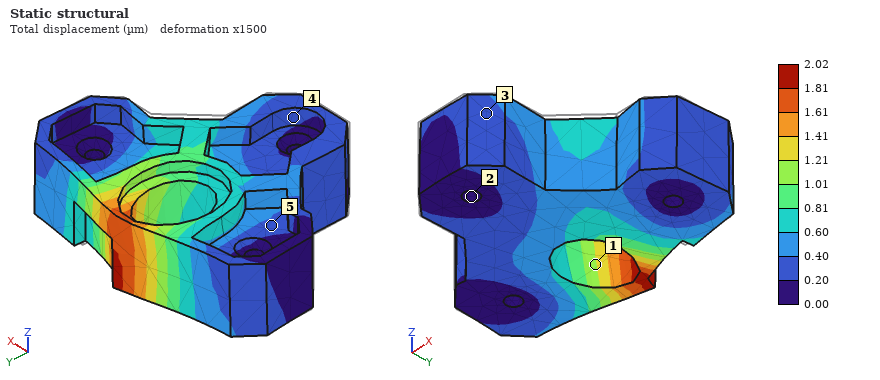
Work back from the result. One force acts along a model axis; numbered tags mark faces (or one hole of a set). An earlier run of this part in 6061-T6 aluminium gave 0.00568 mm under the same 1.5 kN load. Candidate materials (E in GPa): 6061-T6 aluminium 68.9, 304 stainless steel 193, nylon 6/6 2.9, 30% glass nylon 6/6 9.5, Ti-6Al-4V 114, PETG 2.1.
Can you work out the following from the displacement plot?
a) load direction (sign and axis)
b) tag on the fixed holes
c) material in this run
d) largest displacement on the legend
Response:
+Y
2
304 stainless steel
2.02 µm
